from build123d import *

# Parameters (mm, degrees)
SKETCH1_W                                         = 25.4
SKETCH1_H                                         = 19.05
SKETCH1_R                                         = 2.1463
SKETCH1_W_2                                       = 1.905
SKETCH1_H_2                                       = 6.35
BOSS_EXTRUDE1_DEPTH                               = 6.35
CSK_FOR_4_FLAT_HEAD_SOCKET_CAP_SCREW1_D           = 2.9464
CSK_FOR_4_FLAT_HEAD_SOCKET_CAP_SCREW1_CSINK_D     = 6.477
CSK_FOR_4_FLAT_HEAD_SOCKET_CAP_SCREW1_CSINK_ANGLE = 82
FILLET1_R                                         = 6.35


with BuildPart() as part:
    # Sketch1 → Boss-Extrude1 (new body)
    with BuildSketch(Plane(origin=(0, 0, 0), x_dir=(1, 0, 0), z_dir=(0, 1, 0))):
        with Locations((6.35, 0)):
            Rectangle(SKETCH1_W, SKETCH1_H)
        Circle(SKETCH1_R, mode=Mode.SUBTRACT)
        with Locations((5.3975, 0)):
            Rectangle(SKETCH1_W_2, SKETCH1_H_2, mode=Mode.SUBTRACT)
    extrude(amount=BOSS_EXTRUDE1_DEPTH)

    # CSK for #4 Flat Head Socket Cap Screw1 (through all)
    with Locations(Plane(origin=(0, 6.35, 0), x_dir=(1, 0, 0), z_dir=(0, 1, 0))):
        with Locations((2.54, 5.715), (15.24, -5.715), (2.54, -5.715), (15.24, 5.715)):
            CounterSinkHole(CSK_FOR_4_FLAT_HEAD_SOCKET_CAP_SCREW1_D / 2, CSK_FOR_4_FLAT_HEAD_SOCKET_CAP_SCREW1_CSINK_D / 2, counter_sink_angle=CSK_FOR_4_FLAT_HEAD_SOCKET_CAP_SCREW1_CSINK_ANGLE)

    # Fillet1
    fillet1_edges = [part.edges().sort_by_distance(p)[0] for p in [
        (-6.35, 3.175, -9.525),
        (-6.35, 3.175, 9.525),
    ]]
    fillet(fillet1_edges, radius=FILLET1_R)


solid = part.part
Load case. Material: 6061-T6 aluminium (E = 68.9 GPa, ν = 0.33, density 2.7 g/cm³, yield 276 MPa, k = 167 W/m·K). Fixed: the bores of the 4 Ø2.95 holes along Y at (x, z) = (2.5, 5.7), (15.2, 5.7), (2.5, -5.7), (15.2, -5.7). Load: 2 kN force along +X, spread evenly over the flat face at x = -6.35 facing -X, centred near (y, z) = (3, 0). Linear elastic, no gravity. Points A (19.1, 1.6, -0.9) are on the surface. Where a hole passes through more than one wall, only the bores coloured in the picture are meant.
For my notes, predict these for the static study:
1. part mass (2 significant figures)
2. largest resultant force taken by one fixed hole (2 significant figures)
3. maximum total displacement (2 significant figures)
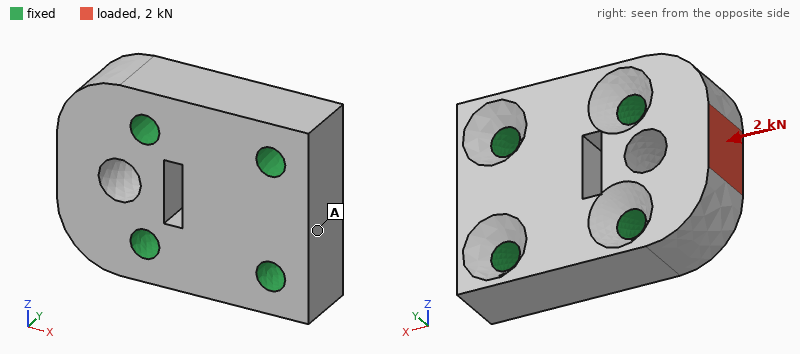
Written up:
6.8 g
1.0 kN
10 µm
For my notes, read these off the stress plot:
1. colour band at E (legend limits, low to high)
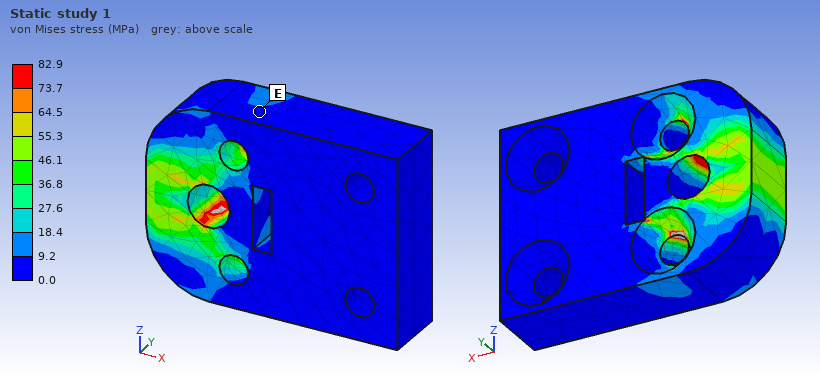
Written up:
0.0 to 9.2 MPa
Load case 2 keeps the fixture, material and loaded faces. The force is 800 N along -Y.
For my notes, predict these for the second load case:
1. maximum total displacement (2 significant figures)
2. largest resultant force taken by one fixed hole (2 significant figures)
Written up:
25 µm
450 N
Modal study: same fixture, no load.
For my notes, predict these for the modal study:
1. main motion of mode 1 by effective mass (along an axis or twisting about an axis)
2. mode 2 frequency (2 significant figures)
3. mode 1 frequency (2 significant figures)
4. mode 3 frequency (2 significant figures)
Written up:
along Y
68 kHz
42 kHz
70 kHz
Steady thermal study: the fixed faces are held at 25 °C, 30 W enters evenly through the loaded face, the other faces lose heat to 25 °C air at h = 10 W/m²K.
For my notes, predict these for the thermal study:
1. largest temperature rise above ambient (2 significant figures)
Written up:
26 K
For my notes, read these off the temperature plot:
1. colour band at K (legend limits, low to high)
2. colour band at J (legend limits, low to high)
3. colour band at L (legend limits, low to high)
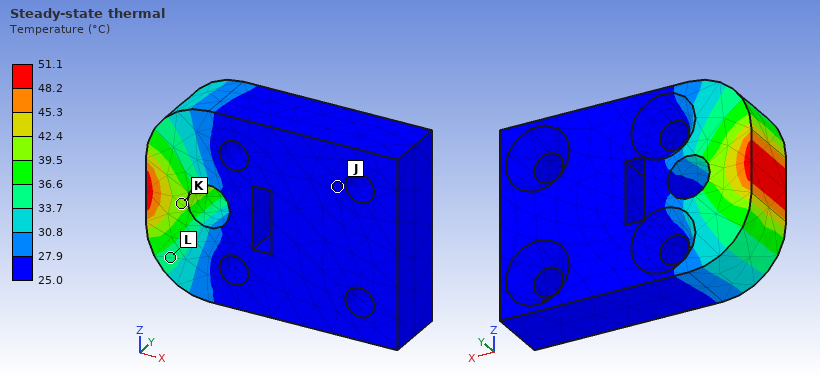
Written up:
39.5 to 42.4 °C
25.0 to 27.9 °C
33.7 to 36.6 °C
